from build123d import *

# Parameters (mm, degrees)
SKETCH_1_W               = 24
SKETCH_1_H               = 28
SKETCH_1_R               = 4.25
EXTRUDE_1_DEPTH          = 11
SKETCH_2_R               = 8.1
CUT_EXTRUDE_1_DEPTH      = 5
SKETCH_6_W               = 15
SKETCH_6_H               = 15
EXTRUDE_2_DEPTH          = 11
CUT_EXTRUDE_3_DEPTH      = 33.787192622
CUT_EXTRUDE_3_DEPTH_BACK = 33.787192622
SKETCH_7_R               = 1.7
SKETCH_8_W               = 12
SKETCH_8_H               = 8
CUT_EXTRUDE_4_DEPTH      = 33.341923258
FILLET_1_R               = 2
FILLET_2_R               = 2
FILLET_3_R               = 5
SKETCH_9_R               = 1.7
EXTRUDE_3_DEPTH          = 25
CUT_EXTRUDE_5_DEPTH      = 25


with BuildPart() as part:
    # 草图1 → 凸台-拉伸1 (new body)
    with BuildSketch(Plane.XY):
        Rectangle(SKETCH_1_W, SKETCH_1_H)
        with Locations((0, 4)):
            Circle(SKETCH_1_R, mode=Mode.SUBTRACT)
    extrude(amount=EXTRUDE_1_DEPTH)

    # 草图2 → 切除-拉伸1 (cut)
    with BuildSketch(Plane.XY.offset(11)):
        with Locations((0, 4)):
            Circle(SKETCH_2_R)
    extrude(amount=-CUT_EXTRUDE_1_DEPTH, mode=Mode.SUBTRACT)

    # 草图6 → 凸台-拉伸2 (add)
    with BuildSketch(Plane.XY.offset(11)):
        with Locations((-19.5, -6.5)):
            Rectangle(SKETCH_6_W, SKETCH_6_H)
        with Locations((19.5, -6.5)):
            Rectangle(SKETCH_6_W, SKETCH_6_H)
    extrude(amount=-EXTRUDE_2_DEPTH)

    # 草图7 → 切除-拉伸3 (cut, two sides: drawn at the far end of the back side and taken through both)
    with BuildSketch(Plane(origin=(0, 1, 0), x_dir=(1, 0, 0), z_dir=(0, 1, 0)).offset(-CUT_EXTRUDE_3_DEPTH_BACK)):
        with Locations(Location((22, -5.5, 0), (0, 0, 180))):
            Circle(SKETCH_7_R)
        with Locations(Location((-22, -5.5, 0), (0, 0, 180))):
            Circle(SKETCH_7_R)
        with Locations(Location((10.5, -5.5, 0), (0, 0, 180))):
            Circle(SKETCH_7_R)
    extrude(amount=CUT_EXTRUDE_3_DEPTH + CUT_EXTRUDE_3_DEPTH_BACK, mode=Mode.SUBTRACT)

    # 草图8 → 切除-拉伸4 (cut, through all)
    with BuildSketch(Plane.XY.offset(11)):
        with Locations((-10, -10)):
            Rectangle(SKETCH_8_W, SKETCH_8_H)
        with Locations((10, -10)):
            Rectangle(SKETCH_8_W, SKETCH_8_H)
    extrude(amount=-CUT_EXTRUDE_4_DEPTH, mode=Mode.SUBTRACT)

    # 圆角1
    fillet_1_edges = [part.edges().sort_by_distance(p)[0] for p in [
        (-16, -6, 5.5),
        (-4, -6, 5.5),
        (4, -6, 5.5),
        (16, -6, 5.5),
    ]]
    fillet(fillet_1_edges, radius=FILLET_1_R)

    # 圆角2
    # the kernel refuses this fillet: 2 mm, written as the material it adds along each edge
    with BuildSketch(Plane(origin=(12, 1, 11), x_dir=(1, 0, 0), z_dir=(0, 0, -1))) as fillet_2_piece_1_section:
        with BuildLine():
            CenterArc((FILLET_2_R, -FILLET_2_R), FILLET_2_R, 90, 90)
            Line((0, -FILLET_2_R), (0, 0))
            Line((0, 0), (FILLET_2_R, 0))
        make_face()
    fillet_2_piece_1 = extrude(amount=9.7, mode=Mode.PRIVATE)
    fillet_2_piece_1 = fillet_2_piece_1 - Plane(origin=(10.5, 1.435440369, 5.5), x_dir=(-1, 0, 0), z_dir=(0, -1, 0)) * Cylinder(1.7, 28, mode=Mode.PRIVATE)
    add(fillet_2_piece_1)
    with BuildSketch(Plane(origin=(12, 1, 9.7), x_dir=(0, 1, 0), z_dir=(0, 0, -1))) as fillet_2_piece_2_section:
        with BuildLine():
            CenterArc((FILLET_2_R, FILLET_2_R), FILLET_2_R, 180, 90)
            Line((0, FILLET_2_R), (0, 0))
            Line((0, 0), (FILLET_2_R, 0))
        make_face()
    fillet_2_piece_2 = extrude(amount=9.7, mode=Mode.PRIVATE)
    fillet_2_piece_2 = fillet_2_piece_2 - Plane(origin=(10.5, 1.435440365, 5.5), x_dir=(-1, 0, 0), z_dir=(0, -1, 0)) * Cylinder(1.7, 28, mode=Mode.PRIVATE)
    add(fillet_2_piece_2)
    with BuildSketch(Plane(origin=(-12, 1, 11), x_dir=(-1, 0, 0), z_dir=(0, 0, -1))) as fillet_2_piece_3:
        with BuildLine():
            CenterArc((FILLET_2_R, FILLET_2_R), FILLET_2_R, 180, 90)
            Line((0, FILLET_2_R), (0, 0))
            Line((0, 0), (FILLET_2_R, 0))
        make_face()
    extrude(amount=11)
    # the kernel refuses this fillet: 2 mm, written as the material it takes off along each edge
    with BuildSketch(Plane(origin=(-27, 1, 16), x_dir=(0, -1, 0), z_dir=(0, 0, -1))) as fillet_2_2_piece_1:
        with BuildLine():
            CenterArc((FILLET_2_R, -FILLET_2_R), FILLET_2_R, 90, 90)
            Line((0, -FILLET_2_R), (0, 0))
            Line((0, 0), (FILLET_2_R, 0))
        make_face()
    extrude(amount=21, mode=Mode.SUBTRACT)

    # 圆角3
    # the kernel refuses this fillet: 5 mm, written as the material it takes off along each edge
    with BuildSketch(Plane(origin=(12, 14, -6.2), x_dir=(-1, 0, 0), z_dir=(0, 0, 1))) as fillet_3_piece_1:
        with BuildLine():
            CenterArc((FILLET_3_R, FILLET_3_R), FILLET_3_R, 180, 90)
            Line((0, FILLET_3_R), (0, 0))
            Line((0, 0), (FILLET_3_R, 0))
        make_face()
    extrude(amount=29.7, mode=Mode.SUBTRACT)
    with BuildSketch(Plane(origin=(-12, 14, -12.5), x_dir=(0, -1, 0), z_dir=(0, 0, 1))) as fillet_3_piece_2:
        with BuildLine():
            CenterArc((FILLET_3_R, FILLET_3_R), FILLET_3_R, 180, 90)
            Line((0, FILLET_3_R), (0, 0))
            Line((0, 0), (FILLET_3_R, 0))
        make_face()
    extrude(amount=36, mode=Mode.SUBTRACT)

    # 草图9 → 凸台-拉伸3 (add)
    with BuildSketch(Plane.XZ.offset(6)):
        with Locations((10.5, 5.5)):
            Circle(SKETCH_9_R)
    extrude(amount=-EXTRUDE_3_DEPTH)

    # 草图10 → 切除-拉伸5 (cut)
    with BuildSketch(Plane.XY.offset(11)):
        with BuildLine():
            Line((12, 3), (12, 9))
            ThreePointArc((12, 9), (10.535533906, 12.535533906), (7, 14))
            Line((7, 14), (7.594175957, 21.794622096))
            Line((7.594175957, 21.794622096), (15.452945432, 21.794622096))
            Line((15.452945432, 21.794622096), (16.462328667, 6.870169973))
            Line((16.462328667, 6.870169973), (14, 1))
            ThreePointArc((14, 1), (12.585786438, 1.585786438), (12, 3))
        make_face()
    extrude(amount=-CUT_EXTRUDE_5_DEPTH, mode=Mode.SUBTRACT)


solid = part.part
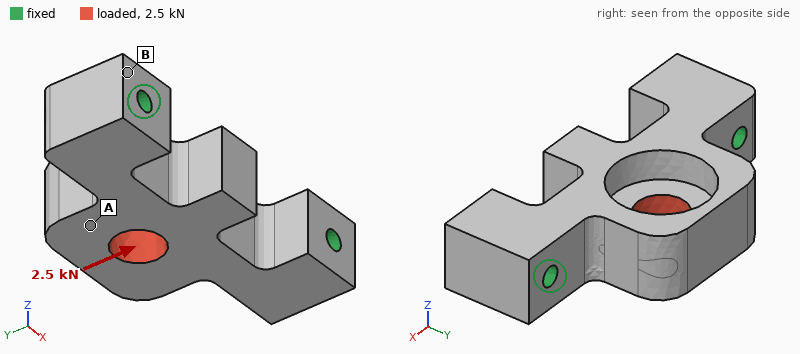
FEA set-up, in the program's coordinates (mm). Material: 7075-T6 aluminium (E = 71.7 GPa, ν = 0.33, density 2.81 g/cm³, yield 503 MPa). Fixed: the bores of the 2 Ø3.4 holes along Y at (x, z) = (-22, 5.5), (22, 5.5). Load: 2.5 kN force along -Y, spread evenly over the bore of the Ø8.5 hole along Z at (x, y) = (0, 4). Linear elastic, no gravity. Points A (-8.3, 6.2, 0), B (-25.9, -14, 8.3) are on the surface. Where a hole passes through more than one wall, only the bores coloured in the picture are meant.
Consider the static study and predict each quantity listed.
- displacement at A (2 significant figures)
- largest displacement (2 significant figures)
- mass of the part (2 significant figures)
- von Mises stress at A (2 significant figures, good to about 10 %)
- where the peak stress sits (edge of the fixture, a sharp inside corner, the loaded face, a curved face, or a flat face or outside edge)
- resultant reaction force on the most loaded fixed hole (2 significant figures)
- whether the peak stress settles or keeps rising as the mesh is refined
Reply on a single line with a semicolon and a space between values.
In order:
22 µm; 31 µm; 24 g; 30 MPa; edge of the fixture; 1.3 kN; keeps rising
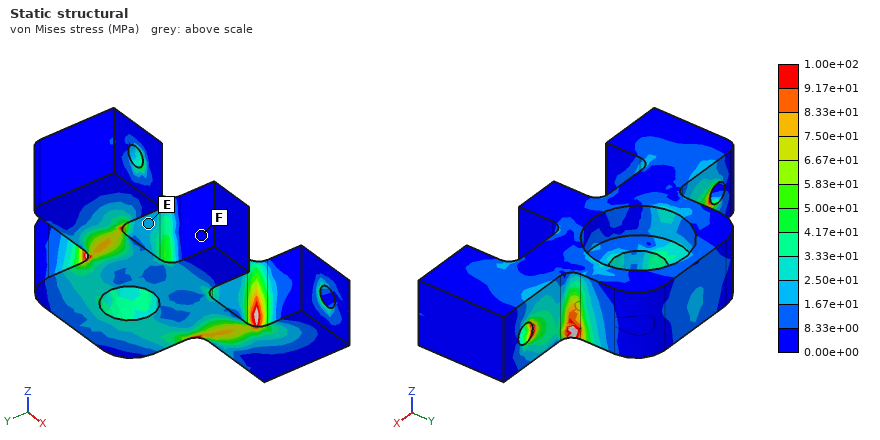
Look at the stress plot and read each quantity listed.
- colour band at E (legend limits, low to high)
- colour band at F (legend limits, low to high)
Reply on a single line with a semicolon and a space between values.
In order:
1.67e+01 to 2.50e+01 MPa; 0.00e+00 to 8.33e+00 MPa
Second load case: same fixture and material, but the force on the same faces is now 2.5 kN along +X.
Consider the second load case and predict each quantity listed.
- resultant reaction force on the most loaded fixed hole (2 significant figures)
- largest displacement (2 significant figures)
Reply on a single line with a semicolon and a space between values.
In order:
1.4 kN; 11 µm
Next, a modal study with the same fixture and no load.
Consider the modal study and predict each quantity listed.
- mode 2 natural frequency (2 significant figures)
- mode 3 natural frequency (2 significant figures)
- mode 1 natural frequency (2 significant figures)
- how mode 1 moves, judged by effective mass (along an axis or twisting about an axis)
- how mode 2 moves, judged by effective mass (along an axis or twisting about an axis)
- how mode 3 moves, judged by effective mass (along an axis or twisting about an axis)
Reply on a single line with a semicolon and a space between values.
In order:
14 kHz; 19 kHz; 10000 Hz; along Z; along Z; along Y
